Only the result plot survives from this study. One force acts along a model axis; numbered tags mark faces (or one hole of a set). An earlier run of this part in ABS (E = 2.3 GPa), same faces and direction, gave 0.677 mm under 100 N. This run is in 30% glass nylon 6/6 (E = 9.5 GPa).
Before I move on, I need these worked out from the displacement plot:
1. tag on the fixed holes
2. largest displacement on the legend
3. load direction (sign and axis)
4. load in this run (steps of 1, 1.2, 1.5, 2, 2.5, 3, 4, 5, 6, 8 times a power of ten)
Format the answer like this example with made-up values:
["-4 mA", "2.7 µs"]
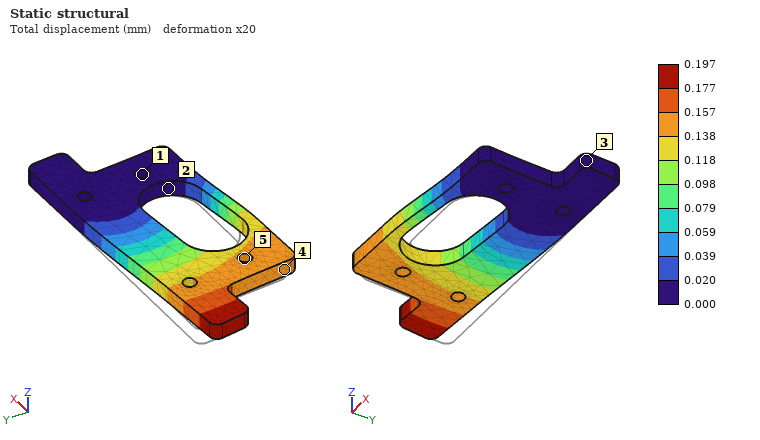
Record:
["1", "0.197 mm", "-Y", "120 N"]
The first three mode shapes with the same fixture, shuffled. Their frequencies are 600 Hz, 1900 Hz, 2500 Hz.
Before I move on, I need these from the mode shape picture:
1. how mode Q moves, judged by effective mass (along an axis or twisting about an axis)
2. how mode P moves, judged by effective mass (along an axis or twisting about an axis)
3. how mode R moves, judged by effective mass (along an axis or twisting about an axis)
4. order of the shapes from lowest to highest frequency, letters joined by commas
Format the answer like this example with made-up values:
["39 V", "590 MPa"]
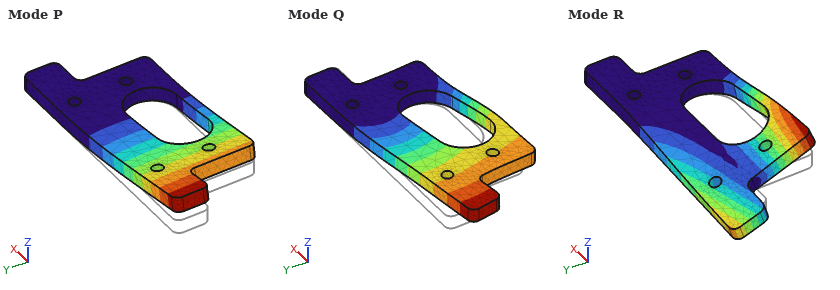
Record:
["along Y", "along Z", "twisting about X", "P, R, Q"]
